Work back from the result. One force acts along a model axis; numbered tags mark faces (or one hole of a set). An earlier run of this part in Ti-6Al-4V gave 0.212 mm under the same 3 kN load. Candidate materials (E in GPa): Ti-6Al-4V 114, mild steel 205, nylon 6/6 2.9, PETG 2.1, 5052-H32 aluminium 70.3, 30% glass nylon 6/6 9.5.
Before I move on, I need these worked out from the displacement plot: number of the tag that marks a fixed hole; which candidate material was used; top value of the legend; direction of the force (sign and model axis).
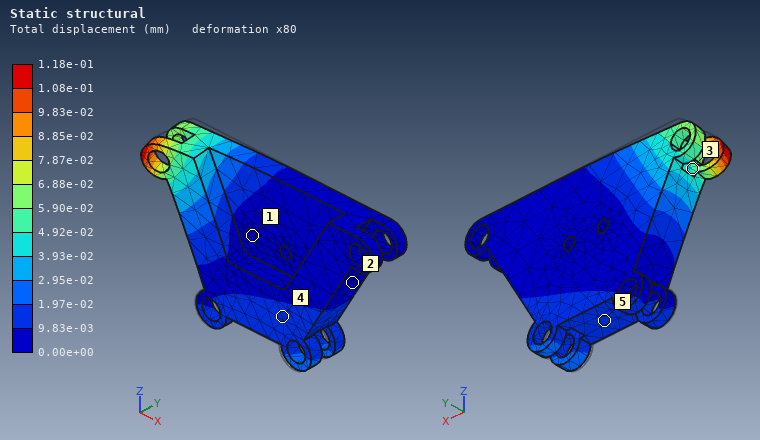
1
mild steel
1.18e-01 mm
-Y
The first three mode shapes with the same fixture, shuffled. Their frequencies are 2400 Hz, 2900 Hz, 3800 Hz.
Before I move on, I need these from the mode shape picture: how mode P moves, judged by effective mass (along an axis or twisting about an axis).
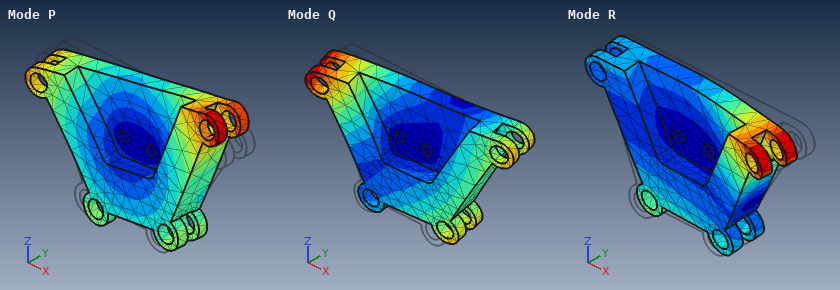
twisting about Y
